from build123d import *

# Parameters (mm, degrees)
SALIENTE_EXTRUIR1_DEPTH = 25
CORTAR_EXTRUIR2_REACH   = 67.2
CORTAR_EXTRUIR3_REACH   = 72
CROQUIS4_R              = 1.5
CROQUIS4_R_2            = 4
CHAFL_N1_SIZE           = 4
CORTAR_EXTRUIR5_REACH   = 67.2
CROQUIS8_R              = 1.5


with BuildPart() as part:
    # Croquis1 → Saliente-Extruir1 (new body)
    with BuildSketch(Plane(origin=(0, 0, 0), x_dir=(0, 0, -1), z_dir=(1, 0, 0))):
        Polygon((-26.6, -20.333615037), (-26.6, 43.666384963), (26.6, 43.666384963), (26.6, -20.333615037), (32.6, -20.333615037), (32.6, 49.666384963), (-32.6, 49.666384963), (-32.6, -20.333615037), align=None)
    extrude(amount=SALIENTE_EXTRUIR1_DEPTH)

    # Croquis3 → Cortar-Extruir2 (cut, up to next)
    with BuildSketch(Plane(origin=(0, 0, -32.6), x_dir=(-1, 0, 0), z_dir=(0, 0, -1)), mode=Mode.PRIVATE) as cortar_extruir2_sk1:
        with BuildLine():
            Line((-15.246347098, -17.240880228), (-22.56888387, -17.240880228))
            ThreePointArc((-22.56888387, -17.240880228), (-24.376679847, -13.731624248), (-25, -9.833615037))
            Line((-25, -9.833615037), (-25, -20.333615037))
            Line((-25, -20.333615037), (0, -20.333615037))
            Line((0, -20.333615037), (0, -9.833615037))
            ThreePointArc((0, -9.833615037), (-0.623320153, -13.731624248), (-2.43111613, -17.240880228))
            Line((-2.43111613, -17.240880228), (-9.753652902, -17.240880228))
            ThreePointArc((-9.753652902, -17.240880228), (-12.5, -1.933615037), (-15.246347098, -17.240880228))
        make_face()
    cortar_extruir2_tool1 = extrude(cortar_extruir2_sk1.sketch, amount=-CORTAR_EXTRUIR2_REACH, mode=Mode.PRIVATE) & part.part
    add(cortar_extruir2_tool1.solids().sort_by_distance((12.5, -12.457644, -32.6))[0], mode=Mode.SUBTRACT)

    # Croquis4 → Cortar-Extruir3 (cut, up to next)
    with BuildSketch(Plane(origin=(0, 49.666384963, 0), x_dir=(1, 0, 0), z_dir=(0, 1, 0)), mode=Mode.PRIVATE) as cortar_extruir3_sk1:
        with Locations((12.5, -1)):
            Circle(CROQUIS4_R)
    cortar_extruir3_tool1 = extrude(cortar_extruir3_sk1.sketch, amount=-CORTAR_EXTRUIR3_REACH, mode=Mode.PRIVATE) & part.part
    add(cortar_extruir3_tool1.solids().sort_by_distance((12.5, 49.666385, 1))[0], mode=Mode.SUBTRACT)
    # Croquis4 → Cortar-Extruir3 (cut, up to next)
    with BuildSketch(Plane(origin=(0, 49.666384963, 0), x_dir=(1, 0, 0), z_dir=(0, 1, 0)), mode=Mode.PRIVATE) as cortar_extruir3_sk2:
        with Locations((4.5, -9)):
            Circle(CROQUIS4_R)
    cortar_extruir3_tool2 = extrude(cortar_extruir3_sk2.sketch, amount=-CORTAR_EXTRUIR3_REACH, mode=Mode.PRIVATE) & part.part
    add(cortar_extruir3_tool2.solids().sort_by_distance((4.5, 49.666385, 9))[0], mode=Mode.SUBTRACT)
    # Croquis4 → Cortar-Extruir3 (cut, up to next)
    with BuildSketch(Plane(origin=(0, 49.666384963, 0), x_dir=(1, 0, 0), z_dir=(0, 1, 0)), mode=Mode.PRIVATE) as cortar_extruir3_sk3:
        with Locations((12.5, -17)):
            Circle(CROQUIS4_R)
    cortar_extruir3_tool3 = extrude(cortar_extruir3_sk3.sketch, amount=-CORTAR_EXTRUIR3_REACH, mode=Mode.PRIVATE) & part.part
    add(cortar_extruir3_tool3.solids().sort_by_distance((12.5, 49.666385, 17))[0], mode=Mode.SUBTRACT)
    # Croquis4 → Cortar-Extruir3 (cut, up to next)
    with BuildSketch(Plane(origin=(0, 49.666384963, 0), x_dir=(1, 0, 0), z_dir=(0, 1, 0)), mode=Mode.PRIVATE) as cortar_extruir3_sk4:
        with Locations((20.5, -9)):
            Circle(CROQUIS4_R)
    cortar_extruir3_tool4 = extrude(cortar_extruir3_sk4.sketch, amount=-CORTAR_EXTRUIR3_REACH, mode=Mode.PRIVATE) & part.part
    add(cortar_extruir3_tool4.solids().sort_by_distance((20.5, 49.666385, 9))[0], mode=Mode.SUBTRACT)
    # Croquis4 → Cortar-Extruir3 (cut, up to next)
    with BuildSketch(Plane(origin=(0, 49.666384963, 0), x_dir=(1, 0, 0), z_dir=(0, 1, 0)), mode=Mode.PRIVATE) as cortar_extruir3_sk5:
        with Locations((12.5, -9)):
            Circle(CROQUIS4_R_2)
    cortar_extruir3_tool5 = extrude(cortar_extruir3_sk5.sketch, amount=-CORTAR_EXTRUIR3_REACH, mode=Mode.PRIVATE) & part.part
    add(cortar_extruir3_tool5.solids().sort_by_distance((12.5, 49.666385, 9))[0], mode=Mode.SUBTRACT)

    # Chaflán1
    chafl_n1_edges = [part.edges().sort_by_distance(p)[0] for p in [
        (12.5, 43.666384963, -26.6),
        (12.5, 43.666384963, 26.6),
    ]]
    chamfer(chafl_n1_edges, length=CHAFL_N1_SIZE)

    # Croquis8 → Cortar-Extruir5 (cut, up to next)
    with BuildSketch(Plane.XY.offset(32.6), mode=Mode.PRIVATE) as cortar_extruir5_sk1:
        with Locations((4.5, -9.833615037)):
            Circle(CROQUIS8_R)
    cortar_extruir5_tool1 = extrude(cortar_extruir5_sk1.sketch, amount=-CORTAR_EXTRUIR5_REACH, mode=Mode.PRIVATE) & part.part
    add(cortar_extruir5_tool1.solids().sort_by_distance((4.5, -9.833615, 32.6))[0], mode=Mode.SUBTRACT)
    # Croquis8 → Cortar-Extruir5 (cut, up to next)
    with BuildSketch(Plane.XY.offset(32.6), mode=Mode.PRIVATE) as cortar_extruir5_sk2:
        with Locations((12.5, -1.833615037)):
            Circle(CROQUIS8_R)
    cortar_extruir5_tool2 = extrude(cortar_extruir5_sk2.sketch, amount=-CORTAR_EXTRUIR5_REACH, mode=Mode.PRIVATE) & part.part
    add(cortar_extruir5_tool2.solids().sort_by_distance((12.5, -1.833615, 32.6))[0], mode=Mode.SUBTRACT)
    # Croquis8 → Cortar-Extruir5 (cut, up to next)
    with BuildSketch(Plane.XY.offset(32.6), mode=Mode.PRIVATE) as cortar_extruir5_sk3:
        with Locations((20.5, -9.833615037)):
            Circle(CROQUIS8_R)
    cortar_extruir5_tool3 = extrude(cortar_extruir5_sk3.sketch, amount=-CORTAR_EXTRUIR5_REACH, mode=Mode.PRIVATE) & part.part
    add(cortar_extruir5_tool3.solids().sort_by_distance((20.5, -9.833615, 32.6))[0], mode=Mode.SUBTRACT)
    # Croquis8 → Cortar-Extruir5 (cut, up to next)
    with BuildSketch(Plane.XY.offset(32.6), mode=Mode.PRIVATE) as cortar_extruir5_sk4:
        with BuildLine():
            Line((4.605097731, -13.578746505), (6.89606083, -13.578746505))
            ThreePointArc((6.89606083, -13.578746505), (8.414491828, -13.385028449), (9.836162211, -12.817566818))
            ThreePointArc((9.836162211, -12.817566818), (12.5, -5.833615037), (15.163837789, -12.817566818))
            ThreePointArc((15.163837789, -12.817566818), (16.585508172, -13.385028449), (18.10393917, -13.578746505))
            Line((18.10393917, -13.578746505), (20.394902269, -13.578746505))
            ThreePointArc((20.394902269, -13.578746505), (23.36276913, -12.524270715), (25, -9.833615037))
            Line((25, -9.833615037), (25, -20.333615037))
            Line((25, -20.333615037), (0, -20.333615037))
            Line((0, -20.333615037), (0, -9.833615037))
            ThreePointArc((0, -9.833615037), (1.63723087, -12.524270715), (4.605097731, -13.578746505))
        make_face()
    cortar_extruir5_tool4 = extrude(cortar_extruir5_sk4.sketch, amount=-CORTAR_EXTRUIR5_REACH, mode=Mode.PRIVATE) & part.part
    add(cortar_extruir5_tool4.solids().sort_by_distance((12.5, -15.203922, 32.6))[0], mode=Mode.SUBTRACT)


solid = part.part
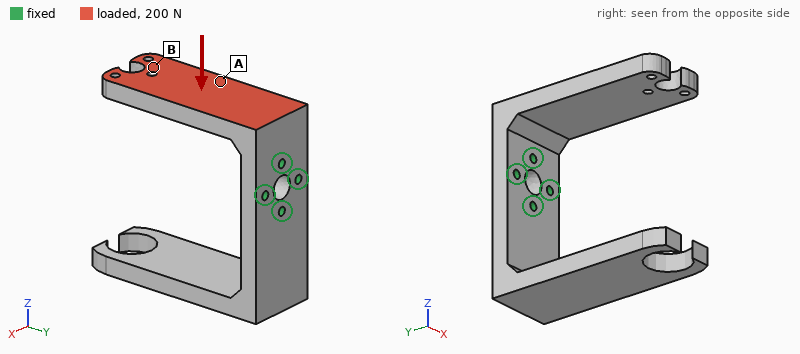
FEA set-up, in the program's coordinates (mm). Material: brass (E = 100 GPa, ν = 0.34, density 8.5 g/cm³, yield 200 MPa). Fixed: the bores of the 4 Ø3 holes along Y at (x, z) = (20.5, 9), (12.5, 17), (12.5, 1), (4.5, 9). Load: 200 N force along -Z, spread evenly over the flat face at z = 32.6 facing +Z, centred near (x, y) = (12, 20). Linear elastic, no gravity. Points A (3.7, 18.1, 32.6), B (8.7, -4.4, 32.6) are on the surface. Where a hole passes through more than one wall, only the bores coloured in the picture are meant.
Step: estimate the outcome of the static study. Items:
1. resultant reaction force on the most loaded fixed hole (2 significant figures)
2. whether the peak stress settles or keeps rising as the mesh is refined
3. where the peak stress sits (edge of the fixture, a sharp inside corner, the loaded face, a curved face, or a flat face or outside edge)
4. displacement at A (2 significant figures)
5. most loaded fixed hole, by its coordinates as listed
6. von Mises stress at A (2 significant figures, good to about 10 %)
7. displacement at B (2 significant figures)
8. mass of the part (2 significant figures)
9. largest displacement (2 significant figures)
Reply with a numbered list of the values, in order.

1. 310 N
2. keeps rising
3. edge of the fixture
4. 0.059 mm
5. (12.5, 17)
6. 9.3 MPa
7. 0.12 mm
8. 220 g
9. 0.15 mm
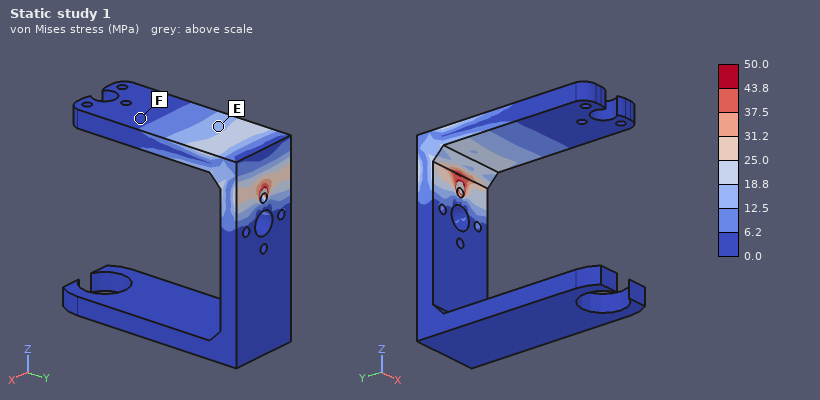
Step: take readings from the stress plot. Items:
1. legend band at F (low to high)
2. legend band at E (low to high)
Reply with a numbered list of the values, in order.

1. 0.0 to 6.2 MPa
2. 12.5 to 18.8 MPa
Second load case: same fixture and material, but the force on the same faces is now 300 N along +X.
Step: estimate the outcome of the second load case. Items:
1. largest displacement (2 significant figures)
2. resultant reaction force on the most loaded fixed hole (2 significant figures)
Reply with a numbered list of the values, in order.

1. 75 µm
2. 330 N
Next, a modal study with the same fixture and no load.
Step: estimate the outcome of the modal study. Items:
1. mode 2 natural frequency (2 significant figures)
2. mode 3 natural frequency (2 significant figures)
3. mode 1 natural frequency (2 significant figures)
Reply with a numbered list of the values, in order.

1. 830 Hz
2. 840 Hz
3. 580 Hz
